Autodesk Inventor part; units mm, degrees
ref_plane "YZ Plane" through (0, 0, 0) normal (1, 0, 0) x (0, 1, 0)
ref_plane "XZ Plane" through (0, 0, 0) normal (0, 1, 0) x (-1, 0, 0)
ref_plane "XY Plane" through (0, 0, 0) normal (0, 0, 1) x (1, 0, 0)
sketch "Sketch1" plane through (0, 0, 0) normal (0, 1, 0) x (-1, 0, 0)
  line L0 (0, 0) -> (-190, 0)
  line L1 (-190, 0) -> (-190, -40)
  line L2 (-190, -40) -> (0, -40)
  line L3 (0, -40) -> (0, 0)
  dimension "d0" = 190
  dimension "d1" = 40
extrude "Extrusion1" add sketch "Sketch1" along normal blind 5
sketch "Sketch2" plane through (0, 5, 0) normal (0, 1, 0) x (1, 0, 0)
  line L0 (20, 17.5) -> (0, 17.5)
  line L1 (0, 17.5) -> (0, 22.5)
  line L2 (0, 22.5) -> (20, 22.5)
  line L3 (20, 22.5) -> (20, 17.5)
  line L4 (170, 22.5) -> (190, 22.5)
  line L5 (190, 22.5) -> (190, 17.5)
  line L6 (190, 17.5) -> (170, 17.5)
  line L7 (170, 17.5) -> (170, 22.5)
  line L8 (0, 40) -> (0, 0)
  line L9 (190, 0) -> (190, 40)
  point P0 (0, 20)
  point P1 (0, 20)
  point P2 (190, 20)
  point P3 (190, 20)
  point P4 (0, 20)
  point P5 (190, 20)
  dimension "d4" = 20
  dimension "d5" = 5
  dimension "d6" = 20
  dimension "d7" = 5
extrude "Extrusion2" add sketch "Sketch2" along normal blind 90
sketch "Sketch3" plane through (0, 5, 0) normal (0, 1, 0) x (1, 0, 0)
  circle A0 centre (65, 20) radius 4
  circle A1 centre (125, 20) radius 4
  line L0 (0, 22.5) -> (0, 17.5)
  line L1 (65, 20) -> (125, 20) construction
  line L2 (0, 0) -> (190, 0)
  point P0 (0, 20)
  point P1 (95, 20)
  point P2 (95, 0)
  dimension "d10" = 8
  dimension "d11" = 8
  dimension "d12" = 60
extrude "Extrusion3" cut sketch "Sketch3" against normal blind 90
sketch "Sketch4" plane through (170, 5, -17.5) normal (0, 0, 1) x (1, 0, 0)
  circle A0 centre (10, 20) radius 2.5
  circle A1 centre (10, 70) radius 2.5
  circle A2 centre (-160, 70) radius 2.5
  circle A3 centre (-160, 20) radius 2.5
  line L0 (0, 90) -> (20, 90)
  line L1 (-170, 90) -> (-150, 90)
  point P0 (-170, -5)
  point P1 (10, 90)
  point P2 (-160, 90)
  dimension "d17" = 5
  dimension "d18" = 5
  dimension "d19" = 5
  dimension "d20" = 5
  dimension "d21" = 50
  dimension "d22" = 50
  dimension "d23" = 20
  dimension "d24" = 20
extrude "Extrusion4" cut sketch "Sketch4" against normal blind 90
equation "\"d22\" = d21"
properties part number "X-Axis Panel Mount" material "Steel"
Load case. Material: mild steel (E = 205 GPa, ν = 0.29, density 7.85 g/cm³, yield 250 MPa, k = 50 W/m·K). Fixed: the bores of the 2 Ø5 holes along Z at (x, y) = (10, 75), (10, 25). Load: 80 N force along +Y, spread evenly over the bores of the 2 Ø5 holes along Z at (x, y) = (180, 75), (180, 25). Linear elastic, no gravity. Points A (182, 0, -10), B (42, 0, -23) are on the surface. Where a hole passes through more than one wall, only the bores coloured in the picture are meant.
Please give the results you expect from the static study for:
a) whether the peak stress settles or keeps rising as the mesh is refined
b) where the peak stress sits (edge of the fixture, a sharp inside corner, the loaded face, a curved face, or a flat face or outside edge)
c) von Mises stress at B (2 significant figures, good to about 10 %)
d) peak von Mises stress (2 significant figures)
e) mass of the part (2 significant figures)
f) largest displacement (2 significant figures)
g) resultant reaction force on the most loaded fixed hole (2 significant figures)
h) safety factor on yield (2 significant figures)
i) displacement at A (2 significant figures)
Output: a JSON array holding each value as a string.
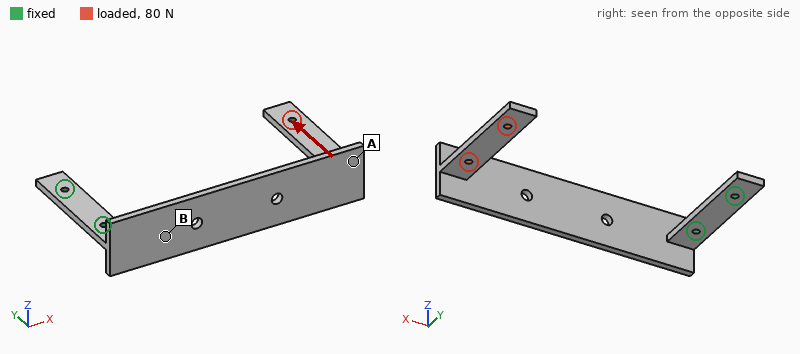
["settles", "a curved face", "63 MPa", "110 MPa", "430 g", "2.1 mm", "180 N", "2.2", "1.6 mm"]
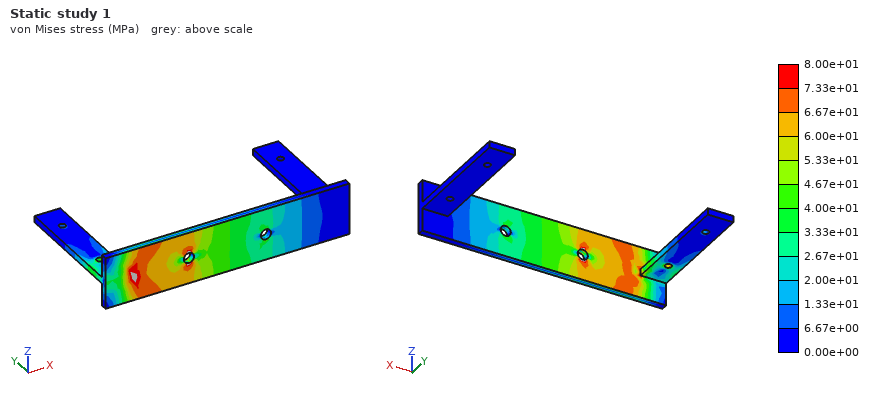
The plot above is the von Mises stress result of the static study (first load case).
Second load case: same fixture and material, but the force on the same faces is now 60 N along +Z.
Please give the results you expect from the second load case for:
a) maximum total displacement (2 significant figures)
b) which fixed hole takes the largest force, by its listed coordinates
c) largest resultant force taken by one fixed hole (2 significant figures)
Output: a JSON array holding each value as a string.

["1.1 mm", "(10, 25)", "58 N"]
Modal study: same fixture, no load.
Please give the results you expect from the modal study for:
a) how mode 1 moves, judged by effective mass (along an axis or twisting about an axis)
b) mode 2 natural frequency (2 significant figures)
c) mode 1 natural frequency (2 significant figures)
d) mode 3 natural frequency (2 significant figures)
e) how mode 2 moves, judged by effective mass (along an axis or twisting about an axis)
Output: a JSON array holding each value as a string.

["along Y", "120 Hz", "89 Hz", "270 Hz", "along Z"]
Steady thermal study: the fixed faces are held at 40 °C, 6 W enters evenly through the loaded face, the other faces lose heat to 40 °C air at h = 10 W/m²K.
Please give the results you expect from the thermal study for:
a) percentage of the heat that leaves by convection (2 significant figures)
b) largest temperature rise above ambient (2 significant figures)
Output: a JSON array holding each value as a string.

["86 %", "67 K"]
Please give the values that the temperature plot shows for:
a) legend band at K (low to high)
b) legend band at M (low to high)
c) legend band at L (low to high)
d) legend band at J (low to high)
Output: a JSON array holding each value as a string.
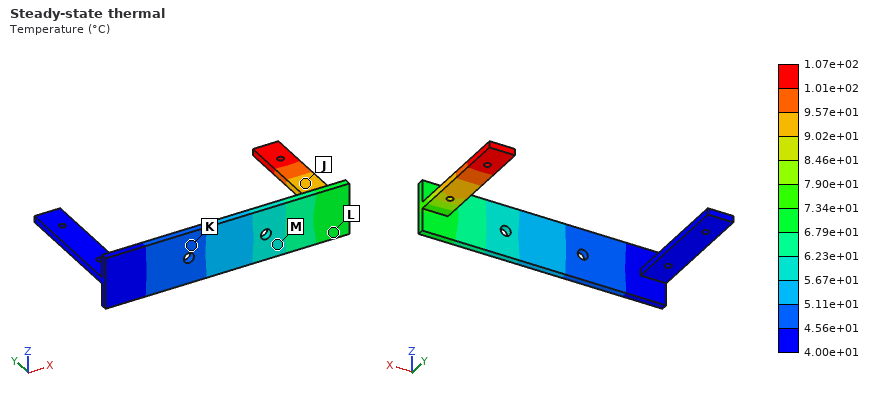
["4.56e+01 to 5.11e+01 °C", "5.67e+01 to 6.23e+01 °C", "6.79e+01 to 7.34e+01 °C", "9.02e+01 to 9.57e+01 °C"]
